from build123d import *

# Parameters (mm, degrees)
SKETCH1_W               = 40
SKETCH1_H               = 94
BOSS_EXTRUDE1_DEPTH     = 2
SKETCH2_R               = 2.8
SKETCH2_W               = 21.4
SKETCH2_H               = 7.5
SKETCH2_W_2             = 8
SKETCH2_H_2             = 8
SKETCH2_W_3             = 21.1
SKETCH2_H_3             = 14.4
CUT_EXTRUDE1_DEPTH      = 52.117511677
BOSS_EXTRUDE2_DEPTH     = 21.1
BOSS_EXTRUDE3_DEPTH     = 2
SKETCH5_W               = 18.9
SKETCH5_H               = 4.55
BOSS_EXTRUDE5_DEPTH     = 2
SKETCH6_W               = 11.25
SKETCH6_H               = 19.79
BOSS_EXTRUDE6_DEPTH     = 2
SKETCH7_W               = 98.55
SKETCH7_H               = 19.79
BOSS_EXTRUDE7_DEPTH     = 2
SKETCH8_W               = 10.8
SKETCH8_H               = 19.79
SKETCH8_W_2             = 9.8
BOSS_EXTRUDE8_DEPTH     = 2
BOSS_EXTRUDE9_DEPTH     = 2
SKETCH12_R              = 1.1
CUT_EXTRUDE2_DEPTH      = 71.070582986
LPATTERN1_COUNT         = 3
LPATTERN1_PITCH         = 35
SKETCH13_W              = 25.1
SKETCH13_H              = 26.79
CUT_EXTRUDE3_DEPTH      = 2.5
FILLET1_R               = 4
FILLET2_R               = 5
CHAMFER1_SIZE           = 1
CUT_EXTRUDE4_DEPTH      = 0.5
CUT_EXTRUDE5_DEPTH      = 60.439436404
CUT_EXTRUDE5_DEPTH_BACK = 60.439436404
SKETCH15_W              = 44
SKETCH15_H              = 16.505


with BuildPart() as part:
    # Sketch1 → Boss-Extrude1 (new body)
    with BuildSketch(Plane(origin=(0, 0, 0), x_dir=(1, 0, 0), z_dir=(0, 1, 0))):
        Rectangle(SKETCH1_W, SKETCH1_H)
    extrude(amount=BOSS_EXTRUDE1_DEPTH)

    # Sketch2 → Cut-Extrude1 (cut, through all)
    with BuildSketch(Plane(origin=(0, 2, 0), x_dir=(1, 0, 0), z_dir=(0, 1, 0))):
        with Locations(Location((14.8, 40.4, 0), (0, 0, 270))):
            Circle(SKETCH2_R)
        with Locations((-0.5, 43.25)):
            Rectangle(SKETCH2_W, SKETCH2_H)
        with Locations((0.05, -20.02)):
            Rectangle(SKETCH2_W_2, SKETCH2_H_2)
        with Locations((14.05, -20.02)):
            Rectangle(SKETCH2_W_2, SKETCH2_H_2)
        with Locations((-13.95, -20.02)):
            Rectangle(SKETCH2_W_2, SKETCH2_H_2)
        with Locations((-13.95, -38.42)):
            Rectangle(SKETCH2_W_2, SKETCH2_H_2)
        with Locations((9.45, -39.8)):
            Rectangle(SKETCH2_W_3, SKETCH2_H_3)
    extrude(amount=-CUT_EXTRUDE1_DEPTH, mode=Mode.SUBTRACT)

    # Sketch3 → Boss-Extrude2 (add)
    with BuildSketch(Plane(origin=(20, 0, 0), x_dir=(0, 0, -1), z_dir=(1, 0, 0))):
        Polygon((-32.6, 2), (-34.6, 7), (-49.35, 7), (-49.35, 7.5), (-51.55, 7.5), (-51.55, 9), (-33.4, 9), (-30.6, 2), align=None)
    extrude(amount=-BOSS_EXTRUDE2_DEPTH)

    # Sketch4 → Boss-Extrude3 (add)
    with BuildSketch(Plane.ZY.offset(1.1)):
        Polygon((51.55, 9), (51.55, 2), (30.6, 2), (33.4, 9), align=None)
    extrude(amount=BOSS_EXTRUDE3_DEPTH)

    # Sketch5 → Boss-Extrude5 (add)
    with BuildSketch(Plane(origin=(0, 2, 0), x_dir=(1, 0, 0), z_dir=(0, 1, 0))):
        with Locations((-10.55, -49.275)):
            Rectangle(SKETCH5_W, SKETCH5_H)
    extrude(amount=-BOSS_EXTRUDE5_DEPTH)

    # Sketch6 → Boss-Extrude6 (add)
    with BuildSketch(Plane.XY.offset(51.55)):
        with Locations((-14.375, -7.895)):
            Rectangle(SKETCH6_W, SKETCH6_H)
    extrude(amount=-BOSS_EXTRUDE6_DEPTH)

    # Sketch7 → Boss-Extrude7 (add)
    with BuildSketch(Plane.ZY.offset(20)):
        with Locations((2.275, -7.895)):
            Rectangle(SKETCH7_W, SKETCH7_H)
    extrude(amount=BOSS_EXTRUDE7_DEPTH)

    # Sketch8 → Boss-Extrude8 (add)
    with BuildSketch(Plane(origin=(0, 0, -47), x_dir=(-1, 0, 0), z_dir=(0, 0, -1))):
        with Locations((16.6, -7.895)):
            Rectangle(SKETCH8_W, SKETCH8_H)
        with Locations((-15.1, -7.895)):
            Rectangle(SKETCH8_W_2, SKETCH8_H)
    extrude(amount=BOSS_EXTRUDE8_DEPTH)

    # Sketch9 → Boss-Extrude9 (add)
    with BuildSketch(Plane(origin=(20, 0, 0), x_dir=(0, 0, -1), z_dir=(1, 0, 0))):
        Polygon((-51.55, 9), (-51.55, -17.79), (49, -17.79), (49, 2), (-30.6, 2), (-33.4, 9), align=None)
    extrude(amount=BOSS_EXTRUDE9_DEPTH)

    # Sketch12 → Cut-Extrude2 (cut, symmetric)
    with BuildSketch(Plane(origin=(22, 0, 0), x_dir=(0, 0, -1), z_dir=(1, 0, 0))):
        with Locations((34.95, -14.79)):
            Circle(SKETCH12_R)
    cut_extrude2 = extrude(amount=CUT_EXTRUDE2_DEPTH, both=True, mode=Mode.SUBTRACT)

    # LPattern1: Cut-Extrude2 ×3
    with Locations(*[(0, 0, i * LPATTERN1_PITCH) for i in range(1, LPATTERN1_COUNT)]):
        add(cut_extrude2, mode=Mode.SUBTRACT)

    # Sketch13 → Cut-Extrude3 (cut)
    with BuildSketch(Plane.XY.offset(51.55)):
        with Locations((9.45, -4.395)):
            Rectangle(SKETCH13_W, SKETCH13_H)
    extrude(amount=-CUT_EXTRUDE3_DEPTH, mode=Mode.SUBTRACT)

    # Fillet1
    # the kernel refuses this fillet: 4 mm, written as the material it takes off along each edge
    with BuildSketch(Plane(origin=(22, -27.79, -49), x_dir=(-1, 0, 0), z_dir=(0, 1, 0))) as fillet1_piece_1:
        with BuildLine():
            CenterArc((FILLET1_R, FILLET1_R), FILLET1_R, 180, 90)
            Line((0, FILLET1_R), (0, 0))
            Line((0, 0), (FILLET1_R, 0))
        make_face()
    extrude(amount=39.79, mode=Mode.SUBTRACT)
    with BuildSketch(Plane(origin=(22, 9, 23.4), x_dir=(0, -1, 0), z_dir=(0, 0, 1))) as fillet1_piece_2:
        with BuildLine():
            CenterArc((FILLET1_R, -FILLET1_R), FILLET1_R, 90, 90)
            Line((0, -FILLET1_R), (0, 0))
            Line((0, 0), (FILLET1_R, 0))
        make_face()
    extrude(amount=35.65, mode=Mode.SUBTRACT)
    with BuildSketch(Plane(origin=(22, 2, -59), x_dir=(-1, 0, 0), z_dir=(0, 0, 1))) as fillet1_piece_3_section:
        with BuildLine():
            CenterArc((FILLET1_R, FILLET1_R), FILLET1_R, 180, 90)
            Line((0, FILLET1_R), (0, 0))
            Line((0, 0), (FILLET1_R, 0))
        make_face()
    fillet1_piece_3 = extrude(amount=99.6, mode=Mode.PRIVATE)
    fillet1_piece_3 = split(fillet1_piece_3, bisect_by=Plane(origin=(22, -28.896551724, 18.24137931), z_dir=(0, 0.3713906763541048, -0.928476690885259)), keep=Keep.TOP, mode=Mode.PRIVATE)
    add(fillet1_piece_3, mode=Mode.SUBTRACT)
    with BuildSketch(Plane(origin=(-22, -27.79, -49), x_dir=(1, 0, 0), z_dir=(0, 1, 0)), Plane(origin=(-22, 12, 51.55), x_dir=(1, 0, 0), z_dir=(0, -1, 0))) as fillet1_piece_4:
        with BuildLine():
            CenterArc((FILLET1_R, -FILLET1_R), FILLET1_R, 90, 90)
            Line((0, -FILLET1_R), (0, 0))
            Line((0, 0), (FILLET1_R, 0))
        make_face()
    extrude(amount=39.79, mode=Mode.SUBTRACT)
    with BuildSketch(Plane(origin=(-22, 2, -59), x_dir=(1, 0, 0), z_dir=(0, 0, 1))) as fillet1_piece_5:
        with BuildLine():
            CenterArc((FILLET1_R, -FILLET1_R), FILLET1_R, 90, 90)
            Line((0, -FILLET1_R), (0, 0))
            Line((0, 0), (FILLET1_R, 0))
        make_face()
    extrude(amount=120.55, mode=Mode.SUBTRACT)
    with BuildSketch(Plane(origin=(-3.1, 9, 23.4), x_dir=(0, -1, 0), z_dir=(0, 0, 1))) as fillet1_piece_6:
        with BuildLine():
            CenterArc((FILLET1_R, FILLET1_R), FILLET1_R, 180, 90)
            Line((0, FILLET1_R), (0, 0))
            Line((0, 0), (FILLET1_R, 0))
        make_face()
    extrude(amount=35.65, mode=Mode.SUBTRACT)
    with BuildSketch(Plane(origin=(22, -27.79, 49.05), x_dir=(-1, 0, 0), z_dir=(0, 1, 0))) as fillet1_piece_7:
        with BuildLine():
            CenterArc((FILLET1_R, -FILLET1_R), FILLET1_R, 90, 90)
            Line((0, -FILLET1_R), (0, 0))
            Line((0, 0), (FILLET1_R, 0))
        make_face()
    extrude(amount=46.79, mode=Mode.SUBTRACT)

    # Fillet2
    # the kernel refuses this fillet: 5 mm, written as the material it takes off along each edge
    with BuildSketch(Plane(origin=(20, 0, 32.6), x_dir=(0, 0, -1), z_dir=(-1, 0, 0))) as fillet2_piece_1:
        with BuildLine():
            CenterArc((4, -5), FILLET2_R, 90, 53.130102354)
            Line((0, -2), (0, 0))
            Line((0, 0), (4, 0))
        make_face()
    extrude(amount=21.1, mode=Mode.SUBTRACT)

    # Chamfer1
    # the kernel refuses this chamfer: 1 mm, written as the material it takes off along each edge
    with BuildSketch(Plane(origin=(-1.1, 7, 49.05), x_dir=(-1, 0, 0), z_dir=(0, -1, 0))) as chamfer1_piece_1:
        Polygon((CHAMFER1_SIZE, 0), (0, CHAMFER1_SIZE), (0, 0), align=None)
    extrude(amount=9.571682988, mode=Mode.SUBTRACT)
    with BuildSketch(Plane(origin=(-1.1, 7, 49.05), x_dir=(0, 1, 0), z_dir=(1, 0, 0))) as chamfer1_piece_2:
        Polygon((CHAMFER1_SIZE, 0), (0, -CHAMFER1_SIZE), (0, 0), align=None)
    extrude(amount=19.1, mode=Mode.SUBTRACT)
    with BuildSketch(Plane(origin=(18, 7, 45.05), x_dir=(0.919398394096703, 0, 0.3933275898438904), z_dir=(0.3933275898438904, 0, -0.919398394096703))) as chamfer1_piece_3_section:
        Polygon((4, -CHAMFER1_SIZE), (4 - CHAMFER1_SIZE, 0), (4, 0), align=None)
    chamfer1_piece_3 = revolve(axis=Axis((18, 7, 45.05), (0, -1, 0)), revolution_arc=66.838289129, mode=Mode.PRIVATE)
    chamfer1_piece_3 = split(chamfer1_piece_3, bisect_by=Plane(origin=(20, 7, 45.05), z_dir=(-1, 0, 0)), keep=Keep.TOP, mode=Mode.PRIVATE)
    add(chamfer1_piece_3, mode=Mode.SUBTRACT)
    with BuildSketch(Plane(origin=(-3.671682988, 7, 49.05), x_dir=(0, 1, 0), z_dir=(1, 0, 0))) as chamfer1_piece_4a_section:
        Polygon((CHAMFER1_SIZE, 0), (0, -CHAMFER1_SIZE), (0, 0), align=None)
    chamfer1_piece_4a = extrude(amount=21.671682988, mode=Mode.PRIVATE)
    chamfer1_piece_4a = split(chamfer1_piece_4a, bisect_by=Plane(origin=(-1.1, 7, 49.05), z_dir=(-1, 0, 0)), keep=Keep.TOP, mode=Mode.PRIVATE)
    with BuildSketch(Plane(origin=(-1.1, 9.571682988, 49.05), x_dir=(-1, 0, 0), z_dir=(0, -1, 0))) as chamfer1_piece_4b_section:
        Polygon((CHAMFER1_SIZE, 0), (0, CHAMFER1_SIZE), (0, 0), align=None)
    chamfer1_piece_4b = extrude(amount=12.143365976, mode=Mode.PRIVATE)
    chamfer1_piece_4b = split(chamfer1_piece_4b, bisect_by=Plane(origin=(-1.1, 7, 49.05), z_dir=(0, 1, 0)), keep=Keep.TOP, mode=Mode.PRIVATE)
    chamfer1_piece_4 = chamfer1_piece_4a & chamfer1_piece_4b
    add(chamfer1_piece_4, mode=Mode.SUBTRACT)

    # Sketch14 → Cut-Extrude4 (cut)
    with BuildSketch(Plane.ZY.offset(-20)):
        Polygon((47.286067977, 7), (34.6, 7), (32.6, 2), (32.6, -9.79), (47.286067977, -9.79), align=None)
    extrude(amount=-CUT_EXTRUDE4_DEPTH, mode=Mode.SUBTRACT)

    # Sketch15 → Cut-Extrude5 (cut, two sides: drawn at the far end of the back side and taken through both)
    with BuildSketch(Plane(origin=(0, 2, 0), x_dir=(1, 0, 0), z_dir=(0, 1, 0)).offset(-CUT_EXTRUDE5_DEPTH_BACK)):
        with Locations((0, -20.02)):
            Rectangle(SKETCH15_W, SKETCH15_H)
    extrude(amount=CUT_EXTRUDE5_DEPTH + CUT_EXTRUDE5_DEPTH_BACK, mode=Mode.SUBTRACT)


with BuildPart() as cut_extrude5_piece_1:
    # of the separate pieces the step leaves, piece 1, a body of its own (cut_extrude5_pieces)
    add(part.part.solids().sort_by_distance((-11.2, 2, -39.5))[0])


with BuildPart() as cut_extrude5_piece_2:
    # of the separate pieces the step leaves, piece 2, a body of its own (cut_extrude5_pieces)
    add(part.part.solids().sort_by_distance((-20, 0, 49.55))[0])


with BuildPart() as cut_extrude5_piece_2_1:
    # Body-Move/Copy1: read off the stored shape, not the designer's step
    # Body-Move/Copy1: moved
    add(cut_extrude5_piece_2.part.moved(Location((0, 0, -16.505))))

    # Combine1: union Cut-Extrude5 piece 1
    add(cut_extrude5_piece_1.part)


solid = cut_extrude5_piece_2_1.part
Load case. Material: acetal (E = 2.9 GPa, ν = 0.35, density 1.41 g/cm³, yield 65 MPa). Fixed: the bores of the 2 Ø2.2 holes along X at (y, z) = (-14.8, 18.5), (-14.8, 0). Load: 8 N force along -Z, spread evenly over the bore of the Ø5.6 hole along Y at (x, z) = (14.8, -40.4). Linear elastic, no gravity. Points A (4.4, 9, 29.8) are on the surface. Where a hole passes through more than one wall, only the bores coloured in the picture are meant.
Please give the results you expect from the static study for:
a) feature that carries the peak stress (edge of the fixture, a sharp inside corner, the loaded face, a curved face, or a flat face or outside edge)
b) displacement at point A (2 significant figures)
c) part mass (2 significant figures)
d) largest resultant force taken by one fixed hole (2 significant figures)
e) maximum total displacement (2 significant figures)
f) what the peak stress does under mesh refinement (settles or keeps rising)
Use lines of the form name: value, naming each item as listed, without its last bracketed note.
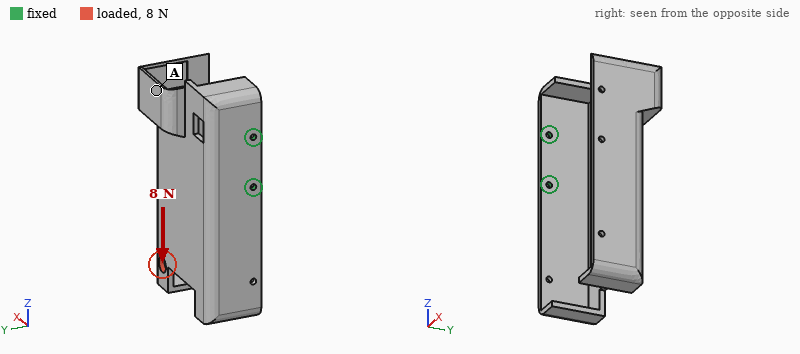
feature that carries the peak stress: edge of the fixture
displacement at point A: 0.48 mm
part mass: 19 g
largest resultant force taken by one fixed hole: 14 N
maximum total displacement: 1.2 mm
what the peak stress does under mesh refinement: keeps rising
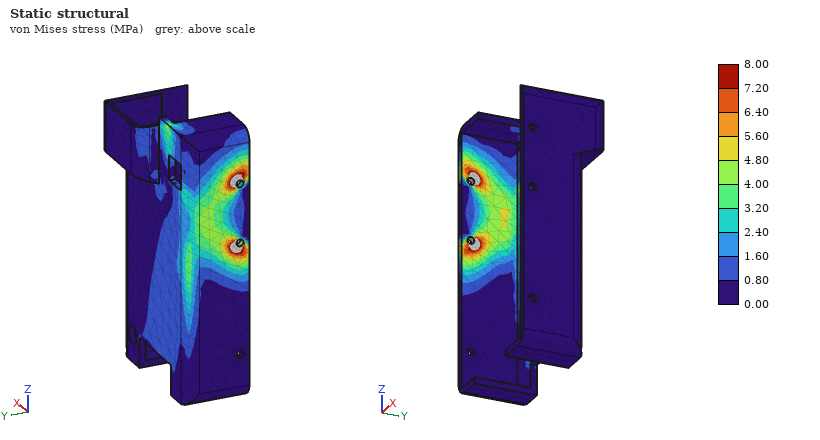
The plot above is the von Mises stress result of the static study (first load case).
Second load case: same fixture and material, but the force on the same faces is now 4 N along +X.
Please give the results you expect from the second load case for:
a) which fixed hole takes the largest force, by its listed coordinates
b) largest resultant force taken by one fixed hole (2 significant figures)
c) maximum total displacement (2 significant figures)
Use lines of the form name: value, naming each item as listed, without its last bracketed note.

which fixed hole takes the largest force, by its listed coordinates: (-14.8, 0)
largest resultant force taken by one fixed hole: 10 N
maximum total displacement: 0.98 mm
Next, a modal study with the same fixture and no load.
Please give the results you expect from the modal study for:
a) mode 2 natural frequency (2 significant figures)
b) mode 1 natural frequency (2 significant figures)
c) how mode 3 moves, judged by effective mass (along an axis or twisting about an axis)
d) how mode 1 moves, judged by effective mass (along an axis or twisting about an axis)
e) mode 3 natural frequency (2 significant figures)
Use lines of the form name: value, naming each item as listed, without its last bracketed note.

mode 2 natural frequency: 130 Hz
mode 1 natural frequency: 84 Hz
how mode 3 moves, judged by effective mass: along X
how mode 1 moves, judged by effective mass: along Y
mode 3 natural frequency: 240 Hz
